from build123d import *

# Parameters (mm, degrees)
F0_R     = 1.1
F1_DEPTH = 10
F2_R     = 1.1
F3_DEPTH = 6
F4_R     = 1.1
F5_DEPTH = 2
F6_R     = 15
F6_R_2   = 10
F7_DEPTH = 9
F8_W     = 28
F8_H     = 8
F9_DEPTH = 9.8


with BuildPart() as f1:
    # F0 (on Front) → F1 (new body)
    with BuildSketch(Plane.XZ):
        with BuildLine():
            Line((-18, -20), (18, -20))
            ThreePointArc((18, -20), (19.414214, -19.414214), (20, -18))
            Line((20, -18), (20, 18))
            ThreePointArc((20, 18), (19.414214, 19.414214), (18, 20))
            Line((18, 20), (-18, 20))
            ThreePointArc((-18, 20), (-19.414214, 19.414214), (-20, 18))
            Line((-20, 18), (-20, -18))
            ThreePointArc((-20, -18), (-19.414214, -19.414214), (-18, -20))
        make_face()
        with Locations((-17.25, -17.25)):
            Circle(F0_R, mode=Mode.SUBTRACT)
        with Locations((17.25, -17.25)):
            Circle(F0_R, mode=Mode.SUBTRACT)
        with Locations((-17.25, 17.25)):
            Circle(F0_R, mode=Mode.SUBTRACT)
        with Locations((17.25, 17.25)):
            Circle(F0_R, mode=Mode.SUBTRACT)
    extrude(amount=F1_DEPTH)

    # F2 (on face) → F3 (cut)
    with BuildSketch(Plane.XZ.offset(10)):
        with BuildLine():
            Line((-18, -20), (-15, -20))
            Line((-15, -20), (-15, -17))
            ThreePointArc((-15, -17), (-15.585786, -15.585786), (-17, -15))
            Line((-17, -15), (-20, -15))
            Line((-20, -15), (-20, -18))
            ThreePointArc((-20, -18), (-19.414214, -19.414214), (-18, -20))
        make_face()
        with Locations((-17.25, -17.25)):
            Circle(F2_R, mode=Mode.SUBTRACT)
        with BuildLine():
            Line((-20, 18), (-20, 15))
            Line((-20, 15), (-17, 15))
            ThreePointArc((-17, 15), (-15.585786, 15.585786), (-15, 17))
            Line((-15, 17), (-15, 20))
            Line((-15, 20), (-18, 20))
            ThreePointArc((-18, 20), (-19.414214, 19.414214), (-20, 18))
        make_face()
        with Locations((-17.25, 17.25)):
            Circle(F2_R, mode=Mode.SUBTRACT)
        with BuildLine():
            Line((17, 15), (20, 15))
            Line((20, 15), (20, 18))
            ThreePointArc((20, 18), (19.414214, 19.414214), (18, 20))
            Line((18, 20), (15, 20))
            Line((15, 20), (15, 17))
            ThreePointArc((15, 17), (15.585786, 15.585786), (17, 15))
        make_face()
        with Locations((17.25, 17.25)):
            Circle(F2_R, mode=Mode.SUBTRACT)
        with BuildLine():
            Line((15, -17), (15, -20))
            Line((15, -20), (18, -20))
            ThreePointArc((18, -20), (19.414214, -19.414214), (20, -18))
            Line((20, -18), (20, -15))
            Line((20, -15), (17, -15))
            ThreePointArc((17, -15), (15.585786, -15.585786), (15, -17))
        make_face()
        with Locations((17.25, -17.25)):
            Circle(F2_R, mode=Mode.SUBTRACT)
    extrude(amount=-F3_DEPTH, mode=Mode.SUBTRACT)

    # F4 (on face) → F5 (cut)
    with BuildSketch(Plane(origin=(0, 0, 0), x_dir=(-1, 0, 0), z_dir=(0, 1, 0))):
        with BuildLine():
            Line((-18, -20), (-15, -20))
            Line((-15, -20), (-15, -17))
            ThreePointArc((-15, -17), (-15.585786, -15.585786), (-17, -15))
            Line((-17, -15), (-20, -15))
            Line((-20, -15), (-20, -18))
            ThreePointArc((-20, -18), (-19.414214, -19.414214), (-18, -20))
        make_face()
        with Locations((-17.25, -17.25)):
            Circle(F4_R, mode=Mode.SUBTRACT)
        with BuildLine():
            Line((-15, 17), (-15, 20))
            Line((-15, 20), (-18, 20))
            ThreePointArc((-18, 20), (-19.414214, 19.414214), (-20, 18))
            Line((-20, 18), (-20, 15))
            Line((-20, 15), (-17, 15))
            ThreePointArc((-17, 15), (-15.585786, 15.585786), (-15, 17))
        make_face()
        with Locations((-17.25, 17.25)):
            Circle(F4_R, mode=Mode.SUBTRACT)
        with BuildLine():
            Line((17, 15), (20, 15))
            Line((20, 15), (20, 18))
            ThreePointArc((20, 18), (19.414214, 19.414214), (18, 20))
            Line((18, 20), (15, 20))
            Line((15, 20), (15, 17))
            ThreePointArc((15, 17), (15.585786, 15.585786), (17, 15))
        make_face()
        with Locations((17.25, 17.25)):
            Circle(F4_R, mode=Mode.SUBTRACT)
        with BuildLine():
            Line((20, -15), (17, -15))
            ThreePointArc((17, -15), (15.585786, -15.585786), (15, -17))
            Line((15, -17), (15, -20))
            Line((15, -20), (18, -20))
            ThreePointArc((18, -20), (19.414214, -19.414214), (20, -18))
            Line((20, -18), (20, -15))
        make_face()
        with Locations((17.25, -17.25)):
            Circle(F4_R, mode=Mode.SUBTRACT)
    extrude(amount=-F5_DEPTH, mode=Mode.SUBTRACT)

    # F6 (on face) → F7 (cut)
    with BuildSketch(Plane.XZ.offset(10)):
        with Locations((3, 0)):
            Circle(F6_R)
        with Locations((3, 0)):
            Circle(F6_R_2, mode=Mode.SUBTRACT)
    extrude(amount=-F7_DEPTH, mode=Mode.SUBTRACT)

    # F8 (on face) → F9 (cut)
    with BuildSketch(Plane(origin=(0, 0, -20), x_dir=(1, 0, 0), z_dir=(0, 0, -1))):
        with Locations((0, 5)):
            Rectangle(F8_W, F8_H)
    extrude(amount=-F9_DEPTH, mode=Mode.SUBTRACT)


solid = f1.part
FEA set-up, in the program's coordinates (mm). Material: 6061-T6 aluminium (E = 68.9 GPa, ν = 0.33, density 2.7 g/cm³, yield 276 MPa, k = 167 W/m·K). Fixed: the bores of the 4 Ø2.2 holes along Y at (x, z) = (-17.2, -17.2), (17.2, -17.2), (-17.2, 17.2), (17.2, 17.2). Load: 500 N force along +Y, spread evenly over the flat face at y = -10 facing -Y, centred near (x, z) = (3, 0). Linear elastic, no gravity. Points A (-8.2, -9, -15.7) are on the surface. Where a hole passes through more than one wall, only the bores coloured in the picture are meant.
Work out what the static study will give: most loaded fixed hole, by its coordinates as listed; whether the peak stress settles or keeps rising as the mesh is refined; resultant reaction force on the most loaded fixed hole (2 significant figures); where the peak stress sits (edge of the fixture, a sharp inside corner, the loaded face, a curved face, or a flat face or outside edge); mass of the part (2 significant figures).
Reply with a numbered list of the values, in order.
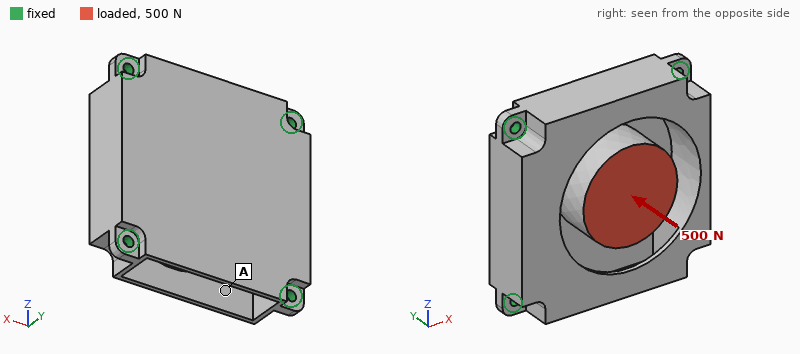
1. (17.2, 17.2)
2. keeps rising
3. 170 N
4. a sharp inside corner
5. 27 g
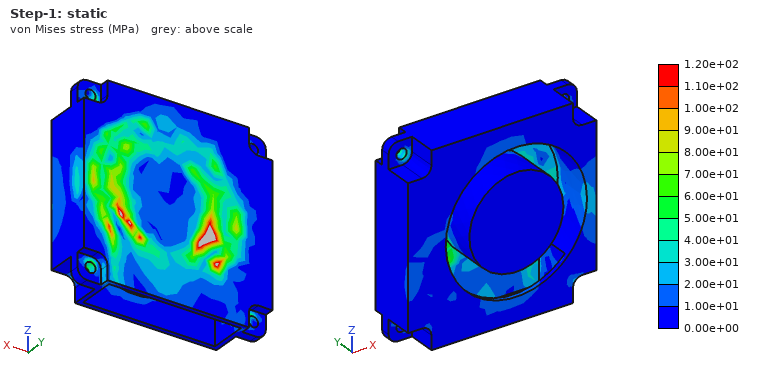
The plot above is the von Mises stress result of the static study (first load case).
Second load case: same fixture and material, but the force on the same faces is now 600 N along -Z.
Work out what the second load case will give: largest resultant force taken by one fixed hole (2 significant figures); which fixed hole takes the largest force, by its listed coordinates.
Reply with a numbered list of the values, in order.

1. 220 N
2. (-17.2, 17.2)
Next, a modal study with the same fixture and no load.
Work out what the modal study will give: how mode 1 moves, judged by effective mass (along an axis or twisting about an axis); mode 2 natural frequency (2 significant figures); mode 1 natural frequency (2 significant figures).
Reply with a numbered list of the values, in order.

1. along Y
2. 7500 Hz
3. 6300 Hz
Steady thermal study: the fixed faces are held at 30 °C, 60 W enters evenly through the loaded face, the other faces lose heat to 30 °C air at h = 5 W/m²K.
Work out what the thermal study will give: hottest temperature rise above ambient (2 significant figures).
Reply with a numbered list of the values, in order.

1. 68 K
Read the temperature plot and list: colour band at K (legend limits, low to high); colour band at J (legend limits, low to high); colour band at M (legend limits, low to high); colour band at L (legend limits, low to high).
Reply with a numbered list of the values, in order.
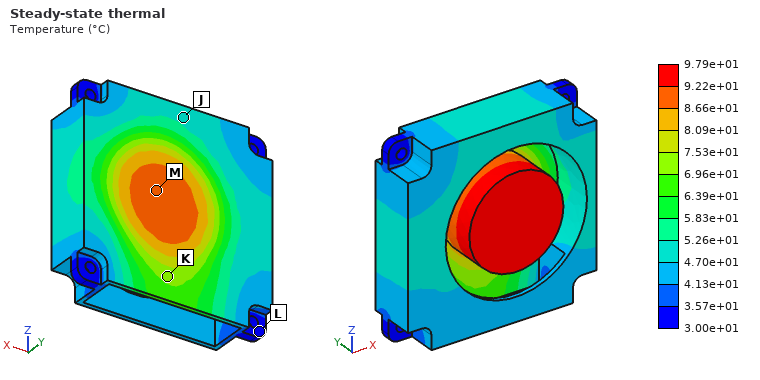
1. 6.96e+01 to 7.53e+01 °C
2. 4.70e+01 to 5.26e+01 °C
3. 8.66e+01 to 9.22e+01 °C
4. 3.00e+01 to 3.57e+01 °C
